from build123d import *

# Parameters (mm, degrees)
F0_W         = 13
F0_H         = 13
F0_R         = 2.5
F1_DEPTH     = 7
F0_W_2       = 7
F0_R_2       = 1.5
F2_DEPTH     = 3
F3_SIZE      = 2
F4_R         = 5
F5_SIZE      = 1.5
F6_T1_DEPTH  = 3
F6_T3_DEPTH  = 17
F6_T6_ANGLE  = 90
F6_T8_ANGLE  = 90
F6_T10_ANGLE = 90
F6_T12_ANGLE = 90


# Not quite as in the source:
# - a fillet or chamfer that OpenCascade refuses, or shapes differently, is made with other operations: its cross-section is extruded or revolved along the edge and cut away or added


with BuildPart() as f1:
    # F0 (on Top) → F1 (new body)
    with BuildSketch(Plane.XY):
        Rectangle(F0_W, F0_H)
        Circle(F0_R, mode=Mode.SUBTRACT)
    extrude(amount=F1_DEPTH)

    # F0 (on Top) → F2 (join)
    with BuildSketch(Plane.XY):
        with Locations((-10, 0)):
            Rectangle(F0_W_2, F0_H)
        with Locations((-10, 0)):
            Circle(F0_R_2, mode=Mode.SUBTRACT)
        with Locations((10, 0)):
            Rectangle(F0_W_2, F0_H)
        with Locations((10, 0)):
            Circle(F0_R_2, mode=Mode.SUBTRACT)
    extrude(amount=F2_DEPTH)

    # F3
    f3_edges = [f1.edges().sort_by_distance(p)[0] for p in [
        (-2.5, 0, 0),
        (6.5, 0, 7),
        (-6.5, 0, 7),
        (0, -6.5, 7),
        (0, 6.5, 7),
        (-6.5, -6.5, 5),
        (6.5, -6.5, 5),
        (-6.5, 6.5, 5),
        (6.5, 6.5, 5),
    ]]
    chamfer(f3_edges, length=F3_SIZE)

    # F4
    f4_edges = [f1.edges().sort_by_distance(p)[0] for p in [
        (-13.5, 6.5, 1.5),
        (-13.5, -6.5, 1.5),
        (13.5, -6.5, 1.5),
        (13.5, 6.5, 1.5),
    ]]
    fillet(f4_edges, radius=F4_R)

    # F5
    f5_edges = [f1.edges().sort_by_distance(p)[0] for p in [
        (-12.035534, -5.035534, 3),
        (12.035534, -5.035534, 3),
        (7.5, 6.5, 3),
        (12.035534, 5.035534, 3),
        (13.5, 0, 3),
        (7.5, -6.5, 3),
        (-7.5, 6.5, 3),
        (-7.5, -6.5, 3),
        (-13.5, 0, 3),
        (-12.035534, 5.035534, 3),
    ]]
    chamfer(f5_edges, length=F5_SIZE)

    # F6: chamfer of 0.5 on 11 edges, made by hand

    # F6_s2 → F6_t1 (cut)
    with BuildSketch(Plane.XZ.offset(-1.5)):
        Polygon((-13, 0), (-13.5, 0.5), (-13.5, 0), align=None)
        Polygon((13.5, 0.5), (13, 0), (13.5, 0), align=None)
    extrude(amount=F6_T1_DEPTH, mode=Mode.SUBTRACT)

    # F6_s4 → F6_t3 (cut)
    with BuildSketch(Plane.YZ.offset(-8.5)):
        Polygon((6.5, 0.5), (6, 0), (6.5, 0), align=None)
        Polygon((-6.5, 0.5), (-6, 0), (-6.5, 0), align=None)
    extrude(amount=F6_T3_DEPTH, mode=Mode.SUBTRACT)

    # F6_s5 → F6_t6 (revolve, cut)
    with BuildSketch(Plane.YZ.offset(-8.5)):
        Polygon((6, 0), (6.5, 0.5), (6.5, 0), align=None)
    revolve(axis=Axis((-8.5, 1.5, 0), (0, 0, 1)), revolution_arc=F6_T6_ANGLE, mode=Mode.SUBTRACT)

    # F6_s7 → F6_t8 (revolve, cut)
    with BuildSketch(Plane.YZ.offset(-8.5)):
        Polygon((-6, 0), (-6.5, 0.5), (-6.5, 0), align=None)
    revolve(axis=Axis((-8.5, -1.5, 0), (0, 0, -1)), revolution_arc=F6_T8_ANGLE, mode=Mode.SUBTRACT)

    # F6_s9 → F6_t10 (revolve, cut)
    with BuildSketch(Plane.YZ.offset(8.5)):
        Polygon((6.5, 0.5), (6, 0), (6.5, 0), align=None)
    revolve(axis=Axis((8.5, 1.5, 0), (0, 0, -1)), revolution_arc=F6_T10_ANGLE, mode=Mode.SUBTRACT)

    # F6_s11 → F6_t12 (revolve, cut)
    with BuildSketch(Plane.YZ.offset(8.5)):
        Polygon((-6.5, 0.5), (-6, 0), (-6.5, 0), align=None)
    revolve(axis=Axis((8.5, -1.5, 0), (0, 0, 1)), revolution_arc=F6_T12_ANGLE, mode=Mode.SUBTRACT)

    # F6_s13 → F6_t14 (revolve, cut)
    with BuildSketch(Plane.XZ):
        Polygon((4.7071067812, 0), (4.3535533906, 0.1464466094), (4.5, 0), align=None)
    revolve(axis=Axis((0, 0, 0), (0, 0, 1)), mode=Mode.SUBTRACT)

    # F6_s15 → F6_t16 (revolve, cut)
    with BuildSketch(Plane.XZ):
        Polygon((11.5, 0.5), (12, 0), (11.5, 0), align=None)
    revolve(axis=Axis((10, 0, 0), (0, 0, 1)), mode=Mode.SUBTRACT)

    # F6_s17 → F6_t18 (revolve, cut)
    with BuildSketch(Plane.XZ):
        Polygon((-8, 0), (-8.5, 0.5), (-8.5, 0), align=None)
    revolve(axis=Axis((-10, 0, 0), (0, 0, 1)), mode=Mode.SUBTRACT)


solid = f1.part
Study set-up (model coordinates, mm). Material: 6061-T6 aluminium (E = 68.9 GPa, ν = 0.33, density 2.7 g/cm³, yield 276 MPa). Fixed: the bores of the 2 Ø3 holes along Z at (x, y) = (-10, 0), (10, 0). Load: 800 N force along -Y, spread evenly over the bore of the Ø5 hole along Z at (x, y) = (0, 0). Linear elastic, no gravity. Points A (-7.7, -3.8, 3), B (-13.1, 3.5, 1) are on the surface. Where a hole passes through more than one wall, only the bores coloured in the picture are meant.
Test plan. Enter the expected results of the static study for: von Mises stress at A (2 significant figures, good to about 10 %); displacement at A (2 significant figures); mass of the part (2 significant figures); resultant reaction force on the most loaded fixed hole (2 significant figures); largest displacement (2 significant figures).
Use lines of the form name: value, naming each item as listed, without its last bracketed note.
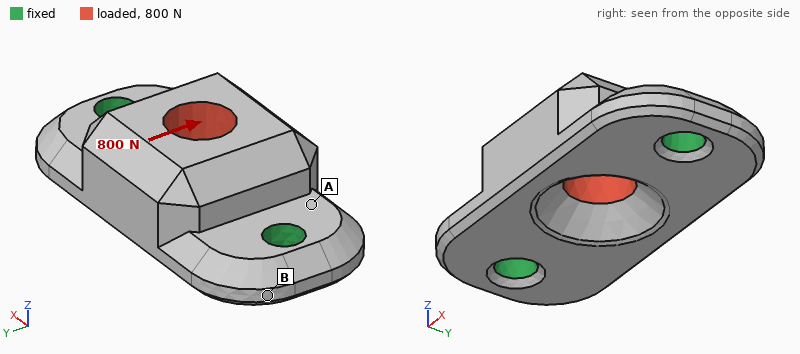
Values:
von Mises stress at A: 42 MPa
displacement at A: 5.7 µm
mass of the part: 3.4 g
resultant reaction force on the most loaded fixed hole: 400 N
largest displacement: 17 µm
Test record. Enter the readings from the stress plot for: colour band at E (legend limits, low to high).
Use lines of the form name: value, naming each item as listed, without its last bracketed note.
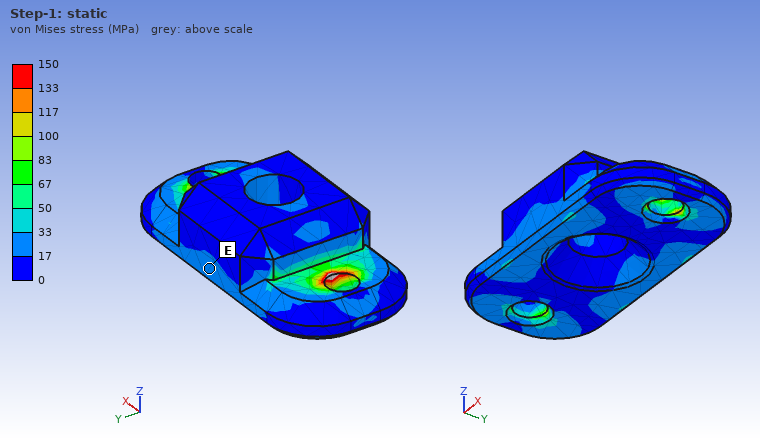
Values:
colour band at E: 17 to 33 MPa
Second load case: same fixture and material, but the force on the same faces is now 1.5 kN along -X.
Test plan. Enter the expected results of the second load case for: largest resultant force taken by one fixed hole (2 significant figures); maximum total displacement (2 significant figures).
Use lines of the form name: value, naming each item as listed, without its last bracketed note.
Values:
largest resultant force taken by one fixed hole: 790 N
maximum total displacement: 6.5 µm
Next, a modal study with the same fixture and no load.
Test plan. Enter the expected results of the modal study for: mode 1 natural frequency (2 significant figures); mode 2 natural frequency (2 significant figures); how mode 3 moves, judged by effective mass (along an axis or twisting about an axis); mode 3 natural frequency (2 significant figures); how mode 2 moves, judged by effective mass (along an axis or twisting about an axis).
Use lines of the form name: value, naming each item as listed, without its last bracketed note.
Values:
mode 1 natural frequency: 24 kHz
mode 2 natural frequency: 34 kHz
how mode 3 moves, judged by effective mass: along Y
mode 3 natural frequency: 53 kHz
how mode 2 moves, judged by effective mass: along Z
